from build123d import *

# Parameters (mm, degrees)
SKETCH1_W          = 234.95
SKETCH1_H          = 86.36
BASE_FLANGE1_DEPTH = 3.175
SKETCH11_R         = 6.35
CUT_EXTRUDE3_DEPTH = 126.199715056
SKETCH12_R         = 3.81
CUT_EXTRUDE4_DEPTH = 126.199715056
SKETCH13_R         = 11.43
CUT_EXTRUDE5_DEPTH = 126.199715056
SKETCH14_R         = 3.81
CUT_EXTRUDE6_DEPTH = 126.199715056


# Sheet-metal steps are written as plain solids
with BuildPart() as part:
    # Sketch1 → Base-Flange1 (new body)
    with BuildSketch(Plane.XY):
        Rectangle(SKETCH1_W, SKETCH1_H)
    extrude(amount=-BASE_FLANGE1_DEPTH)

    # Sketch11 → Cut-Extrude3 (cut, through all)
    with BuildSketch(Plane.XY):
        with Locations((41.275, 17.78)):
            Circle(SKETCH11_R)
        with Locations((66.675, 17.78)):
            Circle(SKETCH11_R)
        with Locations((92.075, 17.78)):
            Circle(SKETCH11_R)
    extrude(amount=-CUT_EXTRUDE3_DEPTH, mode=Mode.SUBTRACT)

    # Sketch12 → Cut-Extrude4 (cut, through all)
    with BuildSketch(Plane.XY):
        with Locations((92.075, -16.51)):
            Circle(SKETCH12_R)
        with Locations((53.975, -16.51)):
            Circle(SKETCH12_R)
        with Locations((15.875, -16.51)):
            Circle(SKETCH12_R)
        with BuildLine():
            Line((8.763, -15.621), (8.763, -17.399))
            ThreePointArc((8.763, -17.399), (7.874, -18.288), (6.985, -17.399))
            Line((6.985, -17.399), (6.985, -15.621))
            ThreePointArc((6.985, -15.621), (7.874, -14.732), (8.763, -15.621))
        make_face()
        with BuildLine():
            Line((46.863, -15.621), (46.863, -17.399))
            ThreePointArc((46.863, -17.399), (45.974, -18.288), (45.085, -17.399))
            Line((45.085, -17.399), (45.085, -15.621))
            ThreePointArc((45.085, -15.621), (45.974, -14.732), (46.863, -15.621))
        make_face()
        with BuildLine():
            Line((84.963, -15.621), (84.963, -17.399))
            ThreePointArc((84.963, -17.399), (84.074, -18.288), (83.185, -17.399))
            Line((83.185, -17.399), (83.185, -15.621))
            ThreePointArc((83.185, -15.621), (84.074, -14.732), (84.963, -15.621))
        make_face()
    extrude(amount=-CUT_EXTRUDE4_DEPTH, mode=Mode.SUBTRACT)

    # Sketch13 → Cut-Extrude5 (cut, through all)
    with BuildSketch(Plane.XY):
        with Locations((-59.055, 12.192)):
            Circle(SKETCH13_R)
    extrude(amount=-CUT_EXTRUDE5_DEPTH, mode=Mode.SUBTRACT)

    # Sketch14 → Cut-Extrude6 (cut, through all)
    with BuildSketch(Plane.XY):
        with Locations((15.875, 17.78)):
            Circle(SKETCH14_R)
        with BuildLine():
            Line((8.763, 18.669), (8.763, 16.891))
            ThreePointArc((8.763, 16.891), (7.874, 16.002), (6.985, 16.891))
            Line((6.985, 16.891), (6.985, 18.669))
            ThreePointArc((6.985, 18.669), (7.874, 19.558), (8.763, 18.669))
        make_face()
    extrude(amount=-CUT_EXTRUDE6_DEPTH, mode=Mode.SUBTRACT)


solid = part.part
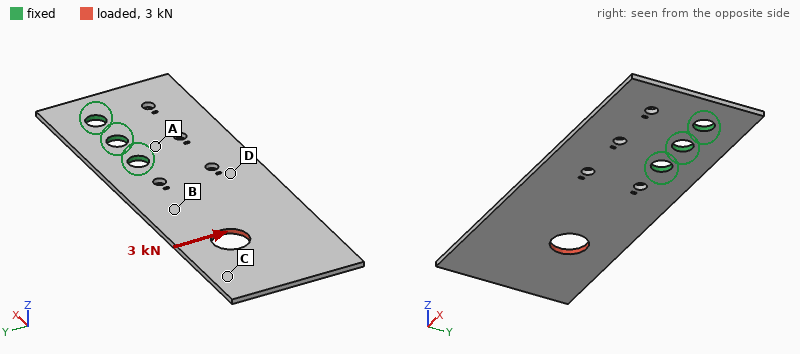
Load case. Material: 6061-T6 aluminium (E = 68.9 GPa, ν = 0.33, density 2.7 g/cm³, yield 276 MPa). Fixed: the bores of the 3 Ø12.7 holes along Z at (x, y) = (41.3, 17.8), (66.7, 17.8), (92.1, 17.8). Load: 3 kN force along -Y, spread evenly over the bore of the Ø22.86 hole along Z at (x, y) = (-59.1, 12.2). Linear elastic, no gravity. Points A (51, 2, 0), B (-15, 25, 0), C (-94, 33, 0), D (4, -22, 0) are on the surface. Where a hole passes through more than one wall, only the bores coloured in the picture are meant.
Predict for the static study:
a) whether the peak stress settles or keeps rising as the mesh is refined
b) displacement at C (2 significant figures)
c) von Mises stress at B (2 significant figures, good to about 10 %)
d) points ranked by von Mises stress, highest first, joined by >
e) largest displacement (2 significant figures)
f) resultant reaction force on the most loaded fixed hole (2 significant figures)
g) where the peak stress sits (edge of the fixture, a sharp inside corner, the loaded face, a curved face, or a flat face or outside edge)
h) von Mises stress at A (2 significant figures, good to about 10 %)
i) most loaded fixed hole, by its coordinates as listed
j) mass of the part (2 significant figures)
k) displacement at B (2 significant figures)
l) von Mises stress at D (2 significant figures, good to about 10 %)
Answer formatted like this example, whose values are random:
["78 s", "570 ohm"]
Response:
["keeps rising", "0.38 mm", "26 MPa", "A > D > B > C", "0.46 mm", "7.7 kN", "edge of the fixture", "54 MPa", "(41.3, 17.8)", "170 g", "0.15 mm", "35 MPa"]
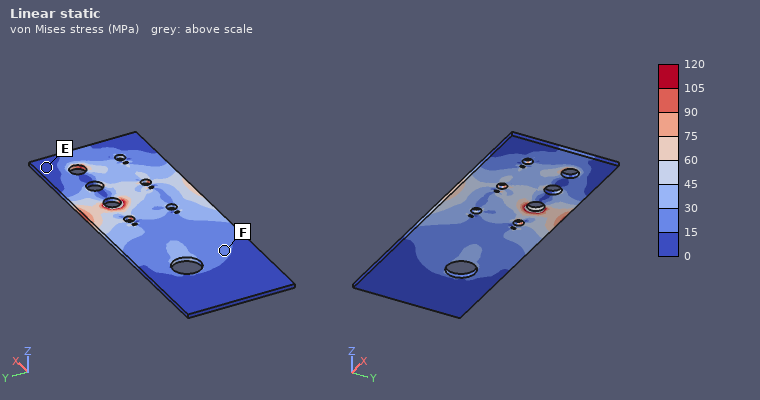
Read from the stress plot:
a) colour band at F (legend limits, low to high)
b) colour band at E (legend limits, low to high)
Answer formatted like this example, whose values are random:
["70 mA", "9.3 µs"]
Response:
["15 to 30 MPa", "0 to 15 MPa"]
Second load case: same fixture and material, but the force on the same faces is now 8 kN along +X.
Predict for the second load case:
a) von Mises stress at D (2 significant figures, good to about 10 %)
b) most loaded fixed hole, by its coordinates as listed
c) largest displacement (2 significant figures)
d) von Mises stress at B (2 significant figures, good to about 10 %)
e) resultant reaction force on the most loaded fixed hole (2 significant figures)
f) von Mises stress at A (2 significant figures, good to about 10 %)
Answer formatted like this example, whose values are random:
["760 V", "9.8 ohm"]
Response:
["16 MPa", "(41.3, 17.8)", "100 µm", "43 MPa", "5.7 kN", "26 MPa"]
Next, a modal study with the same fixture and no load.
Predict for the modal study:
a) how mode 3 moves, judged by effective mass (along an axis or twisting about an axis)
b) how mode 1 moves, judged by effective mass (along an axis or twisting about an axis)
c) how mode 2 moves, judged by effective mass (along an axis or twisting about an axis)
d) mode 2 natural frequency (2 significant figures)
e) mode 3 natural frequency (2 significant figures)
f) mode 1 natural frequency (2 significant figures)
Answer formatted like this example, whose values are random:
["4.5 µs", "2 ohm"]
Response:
["along Z", "along Z", "twisting about X", "350 Hz", "600 Hz", "100 Hz"]
